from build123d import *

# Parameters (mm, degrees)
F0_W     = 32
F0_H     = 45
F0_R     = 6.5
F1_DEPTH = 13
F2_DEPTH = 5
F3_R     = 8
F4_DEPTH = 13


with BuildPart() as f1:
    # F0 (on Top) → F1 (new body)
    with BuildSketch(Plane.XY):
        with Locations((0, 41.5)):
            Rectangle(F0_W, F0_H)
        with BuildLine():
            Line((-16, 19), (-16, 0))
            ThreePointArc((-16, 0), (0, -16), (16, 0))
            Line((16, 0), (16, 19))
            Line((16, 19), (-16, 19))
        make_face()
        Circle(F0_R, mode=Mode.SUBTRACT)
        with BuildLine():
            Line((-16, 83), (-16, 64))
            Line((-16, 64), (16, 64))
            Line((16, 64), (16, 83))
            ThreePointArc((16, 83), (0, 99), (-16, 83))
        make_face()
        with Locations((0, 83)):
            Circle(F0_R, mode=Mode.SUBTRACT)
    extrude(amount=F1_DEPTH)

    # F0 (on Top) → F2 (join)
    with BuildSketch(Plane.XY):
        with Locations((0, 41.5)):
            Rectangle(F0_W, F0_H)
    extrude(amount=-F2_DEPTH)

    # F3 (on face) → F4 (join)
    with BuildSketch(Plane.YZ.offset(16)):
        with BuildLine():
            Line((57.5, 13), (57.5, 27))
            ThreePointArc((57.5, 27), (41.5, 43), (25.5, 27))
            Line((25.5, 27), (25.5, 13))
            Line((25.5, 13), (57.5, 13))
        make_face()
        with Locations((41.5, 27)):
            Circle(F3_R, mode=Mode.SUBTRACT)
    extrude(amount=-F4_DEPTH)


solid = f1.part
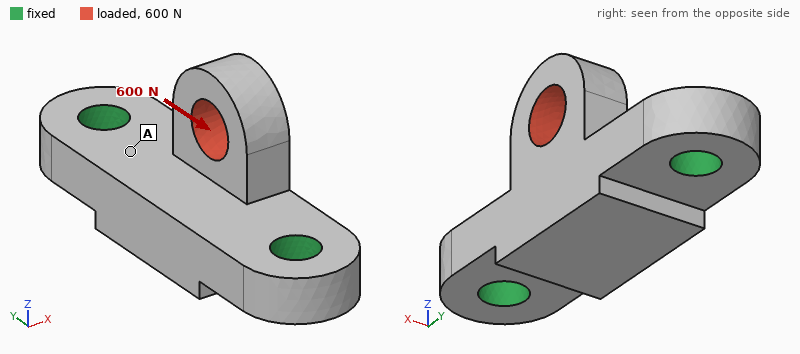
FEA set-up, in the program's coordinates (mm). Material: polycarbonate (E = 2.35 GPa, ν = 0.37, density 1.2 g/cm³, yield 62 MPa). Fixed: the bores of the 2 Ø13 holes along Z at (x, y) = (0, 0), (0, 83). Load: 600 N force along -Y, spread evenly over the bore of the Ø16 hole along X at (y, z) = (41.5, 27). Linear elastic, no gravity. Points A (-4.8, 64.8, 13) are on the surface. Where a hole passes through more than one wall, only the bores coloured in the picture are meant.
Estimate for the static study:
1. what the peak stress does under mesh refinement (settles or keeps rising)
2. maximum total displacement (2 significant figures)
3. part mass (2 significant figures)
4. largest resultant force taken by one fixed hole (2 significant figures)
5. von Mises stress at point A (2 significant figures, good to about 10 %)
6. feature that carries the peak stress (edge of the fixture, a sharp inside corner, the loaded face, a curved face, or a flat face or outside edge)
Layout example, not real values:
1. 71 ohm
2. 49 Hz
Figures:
1. keeps rising
2. 0.20 mm
3. 69 g
4. 370 N
5. 1.6 MPa
6. a sharp inside corner
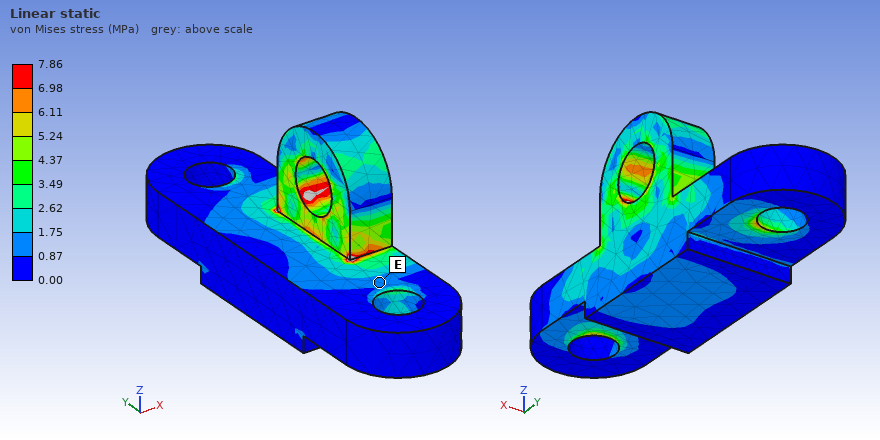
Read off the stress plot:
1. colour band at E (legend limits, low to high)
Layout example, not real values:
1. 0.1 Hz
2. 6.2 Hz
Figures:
1. 0.87 to 1.75 MPa
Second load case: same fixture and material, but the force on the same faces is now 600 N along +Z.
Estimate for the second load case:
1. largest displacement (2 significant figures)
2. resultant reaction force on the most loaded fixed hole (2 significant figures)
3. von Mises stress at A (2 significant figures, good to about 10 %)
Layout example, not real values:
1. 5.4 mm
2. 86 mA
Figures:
1. 0.19 mm
2. 300 N
3. 1.8 MPa
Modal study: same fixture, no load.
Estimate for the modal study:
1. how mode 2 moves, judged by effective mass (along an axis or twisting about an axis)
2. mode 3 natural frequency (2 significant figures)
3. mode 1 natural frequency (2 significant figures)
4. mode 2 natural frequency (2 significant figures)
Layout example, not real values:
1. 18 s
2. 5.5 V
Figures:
1. along Z
2. 3100 Hz
3. 1700 Hz
4. 2600 Hz
